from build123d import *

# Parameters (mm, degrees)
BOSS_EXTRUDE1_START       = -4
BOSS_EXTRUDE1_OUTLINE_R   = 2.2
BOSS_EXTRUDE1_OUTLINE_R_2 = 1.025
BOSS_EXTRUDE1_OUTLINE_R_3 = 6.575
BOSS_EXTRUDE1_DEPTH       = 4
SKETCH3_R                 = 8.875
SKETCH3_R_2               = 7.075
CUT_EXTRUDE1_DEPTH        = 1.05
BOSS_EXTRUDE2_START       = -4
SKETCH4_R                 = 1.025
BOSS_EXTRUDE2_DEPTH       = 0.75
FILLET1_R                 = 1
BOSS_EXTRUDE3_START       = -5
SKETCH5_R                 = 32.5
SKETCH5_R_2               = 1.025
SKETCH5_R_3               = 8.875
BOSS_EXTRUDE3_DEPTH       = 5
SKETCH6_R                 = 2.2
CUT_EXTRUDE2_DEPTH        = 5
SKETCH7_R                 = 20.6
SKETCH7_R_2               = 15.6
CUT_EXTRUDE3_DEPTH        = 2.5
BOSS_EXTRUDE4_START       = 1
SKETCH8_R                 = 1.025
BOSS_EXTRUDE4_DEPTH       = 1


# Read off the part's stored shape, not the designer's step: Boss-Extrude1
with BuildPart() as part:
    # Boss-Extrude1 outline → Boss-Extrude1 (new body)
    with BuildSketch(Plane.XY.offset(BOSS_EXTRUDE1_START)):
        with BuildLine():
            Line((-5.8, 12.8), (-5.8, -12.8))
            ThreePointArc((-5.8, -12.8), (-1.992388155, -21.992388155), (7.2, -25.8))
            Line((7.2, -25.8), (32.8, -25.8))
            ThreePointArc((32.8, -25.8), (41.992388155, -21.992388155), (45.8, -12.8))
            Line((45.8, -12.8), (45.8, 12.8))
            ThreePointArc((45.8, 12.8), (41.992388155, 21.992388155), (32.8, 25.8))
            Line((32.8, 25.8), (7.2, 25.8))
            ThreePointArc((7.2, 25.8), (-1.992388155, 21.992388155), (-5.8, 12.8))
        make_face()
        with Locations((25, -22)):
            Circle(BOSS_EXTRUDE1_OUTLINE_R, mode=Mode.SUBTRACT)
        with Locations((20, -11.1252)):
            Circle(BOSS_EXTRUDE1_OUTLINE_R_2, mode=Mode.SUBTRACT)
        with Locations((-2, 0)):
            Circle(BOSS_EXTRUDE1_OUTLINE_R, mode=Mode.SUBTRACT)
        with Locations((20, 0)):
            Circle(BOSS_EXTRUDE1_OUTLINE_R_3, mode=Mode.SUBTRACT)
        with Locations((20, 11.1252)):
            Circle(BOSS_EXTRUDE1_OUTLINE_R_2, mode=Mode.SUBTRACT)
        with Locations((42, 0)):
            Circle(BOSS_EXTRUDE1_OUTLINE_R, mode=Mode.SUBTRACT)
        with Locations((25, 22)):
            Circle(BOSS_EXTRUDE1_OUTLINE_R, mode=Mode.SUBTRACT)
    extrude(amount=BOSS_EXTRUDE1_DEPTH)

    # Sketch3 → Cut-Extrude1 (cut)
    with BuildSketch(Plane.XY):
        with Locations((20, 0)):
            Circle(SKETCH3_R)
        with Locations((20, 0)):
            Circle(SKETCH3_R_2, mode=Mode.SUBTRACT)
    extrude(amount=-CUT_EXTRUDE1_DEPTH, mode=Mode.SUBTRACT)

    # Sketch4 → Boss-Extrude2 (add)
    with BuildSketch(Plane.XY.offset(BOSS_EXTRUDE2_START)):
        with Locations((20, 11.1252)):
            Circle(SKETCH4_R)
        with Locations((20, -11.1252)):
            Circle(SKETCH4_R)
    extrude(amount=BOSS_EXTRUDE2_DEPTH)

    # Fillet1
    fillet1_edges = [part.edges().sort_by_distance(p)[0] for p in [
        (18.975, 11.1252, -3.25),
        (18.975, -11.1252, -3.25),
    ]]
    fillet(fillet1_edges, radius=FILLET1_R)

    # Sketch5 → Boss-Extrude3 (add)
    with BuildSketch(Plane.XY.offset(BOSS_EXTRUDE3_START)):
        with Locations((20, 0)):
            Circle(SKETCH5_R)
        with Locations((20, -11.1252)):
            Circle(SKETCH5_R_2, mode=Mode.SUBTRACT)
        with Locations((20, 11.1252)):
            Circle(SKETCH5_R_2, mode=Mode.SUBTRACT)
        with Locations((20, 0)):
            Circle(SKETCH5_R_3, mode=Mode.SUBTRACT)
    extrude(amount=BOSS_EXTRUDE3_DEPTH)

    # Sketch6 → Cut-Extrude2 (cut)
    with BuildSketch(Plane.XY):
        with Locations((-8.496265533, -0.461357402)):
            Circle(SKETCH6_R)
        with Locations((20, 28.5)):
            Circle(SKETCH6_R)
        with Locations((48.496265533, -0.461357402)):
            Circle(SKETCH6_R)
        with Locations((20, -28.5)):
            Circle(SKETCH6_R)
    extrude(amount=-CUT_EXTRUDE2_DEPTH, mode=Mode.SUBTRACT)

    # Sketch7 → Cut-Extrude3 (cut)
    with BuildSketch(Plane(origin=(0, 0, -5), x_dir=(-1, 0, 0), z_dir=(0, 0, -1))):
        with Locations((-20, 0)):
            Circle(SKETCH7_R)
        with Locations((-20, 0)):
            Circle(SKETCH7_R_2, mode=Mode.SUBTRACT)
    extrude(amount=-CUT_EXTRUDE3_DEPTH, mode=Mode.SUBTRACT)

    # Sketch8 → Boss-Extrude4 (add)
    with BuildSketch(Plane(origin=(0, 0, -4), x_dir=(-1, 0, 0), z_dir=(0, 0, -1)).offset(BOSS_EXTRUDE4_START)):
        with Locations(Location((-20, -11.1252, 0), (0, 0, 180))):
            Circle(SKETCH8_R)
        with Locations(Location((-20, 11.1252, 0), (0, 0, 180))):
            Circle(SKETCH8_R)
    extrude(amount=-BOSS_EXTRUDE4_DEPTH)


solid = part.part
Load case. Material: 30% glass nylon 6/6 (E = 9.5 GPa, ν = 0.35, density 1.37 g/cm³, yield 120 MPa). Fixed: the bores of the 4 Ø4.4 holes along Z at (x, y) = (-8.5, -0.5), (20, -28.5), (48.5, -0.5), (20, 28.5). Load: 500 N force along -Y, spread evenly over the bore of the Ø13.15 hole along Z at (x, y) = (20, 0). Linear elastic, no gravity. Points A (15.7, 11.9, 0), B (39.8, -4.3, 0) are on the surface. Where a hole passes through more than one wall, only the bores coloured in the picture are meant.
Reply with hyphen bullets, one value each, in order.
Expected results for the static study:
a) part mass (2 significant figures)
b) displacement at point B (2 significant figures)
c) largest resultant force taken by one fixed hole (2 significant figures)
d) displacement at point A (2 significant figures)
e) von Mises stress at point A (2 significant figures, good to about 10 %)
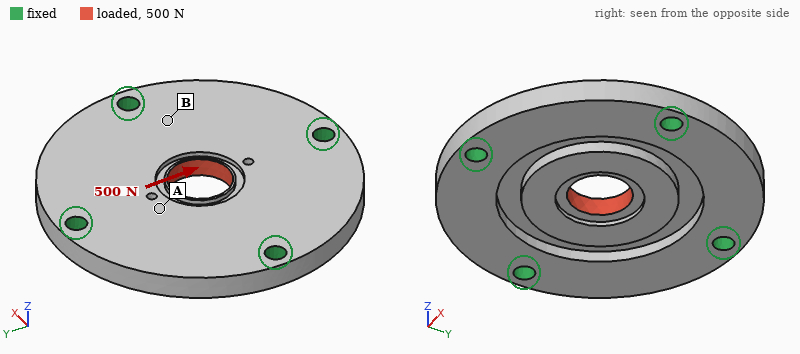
- 19 g
- 2.7 µm
- 150 N
- 5.9 µm
- 2.9 MPa
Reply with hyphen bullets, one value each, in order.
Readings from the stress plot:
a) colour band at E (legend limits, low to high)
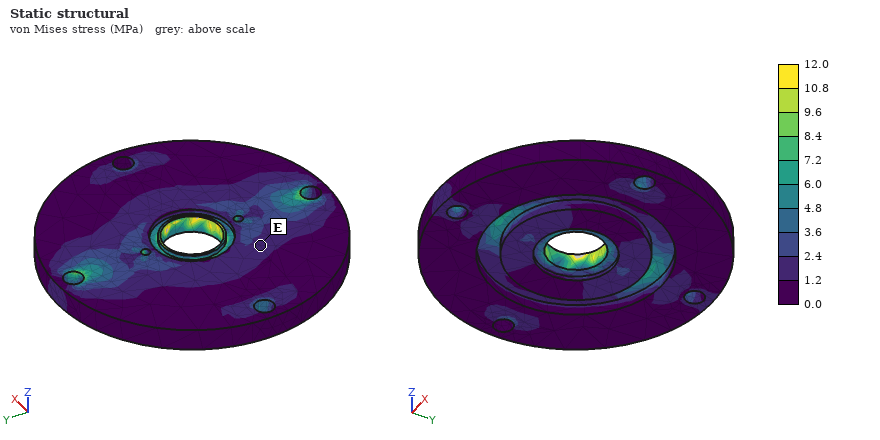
- 1.2 to 2.4 MPa
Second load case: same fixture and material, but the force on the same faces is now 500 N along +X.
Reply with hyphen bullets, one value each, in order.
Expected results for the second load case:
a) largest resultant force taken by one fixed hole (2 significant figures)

- 150 N
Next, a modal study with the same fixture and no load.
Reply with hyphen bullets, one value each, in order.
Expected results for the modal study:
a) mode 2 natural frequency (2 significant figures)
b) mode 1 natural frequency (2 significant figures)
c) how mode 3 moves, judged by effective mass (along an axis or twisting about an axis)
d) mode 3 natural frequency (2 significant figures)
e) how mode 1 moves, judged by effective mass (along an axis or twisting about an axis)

- 6600 Hz
- 5700 Hz
- twisting about X
- 6900 Hz
- along Z
